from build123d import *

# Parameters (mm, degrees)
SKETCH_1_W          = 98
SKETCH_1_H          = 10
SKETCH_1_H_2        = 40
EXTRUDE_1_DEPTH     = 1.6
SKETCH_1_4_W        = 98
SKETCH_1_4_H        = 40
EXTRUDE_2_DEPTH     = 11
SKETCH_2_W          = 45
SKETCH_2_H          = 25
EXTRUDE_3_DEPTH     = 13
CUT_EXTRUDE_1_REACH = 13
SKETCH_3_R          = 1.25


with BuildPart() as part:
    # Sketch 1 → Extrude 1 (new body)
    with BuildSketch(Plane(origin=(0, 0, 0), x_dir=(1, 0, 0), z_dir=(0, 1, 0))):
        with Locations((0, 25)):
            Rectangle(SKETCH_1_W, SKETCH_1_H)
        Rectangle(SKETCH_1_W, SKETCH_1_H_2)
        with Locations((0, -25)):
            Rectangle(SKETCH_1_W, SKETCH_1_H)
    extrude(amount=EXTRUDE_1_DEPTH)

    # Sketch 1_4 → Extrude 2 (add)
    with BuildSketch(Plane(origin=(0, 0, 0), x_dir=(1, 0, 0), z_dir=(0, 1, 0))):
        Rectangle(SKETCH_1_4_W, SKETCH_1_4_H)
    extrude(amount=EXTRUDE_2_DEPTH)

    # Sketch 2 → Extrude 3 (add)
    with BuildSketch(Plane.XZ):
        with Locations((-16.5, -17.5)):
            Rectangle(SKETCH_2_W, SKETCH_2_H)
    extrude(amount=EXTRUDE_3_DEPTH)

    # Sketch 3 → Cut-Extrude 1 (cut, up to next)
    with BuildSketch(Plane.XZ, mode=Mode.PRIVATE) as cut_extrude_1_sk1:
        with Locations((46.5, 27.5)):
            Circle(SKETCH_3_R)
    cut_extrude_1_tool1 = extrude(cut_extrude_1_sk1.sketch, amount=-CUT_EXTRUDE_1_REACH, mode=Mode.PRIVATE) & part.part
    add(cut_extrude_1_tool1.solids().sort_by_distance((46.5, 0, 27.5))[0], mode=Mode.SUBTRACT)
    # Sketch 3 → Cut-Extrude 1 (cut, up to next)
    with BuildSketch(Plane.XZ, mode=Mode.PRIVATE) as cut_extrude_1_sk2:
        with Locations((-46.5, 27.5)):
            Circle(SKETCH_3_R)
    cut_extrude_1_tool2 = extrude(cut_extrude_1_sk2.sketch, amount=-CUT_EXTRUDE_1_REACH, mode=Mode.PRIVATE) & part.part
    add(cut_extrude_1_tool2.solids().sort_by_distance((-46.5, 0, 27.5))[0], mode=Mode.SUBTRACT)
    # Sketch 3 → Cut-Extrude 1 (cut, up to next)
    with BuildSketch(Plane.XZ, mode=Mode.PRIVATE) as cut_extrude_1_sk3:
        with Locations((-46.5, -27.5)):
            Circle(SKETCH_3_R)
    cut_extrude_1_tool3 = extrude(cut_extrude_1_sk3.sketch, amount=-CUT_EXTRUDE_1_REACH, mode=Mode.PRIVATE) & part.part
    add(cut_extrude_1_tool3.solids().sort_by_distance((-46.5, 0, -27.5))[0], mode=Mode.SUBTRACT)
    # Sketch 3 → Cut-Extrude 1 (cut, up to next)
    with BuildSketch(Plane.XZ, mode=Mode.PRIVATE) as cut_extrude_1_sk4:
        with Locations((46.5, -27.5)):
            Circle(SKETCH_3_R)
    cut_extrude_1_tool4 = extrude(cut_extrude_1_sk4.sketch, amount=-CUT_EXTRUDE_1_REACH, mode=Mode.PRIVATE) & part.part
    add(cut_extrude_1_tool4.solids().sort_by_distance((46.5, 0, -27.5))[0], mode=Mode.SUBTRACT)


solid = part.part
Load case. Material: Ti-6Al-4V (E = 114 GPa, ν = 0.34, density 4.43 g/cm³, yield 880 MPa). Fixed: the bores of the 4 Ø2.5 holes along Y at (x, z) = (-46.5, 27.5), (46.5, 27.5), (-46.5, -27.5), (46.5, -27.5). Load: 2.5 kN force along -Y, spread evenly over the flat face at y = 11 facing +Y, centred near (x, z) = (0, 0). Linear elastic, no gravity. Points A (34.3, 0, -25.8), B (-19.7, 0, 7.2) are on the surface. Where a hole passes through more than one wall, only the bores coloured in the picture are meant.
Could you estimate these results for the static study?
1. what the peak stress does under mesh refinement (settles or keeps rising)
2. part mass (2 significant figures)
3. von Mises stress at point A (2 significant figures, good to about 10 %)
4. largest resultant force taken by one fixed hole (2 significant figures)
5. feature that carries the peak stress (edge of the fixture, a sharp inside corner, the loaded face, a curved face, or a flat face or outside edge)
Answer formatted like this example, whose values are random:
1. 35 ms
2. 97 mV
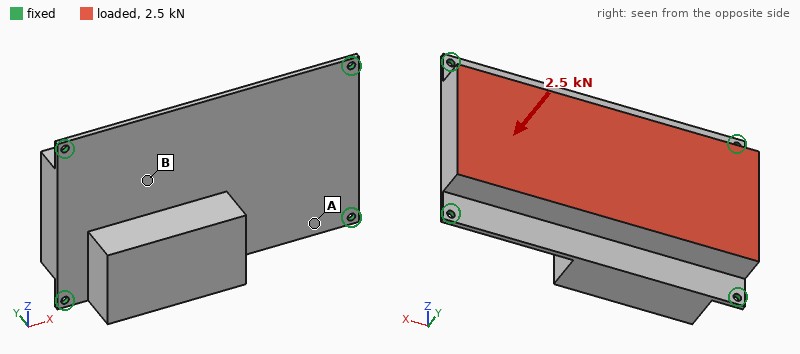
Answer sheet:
1. keeps rising
2. 270 g
3. 62 MPa
4. 860 N
5. edge of the fixture
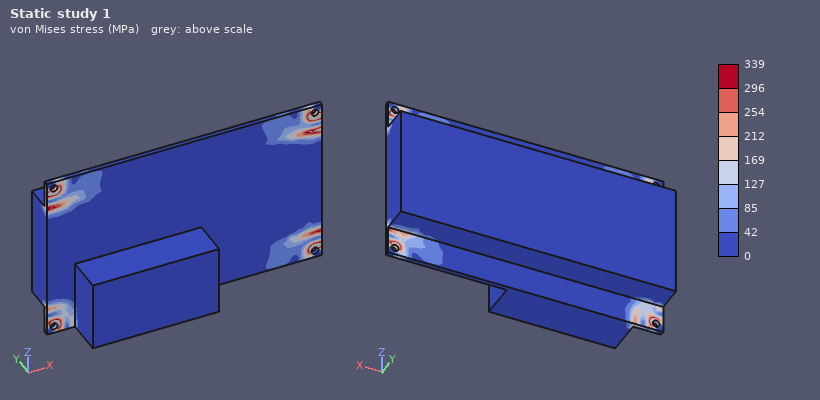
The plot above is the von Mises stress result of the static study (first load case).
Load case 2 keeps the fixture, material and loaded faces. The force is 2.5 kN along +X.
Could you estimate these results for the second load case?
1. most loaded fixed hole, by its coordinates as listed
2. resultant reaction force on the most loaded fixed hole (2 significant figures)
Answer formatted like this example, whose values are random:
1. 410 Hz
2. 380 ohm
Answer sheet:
1. (-46.5, -27.5)
2. 790 N
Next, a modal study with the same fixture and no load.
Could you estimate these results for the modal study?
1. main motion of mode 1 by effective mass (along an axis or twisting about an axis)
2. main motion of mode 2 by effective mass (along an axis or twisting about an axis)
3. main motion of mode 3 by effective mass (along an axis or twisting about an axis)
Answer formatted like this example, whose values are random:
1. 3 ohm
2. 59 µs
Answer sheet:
1. along Y
2. twisting about X
3. twisting about Z
